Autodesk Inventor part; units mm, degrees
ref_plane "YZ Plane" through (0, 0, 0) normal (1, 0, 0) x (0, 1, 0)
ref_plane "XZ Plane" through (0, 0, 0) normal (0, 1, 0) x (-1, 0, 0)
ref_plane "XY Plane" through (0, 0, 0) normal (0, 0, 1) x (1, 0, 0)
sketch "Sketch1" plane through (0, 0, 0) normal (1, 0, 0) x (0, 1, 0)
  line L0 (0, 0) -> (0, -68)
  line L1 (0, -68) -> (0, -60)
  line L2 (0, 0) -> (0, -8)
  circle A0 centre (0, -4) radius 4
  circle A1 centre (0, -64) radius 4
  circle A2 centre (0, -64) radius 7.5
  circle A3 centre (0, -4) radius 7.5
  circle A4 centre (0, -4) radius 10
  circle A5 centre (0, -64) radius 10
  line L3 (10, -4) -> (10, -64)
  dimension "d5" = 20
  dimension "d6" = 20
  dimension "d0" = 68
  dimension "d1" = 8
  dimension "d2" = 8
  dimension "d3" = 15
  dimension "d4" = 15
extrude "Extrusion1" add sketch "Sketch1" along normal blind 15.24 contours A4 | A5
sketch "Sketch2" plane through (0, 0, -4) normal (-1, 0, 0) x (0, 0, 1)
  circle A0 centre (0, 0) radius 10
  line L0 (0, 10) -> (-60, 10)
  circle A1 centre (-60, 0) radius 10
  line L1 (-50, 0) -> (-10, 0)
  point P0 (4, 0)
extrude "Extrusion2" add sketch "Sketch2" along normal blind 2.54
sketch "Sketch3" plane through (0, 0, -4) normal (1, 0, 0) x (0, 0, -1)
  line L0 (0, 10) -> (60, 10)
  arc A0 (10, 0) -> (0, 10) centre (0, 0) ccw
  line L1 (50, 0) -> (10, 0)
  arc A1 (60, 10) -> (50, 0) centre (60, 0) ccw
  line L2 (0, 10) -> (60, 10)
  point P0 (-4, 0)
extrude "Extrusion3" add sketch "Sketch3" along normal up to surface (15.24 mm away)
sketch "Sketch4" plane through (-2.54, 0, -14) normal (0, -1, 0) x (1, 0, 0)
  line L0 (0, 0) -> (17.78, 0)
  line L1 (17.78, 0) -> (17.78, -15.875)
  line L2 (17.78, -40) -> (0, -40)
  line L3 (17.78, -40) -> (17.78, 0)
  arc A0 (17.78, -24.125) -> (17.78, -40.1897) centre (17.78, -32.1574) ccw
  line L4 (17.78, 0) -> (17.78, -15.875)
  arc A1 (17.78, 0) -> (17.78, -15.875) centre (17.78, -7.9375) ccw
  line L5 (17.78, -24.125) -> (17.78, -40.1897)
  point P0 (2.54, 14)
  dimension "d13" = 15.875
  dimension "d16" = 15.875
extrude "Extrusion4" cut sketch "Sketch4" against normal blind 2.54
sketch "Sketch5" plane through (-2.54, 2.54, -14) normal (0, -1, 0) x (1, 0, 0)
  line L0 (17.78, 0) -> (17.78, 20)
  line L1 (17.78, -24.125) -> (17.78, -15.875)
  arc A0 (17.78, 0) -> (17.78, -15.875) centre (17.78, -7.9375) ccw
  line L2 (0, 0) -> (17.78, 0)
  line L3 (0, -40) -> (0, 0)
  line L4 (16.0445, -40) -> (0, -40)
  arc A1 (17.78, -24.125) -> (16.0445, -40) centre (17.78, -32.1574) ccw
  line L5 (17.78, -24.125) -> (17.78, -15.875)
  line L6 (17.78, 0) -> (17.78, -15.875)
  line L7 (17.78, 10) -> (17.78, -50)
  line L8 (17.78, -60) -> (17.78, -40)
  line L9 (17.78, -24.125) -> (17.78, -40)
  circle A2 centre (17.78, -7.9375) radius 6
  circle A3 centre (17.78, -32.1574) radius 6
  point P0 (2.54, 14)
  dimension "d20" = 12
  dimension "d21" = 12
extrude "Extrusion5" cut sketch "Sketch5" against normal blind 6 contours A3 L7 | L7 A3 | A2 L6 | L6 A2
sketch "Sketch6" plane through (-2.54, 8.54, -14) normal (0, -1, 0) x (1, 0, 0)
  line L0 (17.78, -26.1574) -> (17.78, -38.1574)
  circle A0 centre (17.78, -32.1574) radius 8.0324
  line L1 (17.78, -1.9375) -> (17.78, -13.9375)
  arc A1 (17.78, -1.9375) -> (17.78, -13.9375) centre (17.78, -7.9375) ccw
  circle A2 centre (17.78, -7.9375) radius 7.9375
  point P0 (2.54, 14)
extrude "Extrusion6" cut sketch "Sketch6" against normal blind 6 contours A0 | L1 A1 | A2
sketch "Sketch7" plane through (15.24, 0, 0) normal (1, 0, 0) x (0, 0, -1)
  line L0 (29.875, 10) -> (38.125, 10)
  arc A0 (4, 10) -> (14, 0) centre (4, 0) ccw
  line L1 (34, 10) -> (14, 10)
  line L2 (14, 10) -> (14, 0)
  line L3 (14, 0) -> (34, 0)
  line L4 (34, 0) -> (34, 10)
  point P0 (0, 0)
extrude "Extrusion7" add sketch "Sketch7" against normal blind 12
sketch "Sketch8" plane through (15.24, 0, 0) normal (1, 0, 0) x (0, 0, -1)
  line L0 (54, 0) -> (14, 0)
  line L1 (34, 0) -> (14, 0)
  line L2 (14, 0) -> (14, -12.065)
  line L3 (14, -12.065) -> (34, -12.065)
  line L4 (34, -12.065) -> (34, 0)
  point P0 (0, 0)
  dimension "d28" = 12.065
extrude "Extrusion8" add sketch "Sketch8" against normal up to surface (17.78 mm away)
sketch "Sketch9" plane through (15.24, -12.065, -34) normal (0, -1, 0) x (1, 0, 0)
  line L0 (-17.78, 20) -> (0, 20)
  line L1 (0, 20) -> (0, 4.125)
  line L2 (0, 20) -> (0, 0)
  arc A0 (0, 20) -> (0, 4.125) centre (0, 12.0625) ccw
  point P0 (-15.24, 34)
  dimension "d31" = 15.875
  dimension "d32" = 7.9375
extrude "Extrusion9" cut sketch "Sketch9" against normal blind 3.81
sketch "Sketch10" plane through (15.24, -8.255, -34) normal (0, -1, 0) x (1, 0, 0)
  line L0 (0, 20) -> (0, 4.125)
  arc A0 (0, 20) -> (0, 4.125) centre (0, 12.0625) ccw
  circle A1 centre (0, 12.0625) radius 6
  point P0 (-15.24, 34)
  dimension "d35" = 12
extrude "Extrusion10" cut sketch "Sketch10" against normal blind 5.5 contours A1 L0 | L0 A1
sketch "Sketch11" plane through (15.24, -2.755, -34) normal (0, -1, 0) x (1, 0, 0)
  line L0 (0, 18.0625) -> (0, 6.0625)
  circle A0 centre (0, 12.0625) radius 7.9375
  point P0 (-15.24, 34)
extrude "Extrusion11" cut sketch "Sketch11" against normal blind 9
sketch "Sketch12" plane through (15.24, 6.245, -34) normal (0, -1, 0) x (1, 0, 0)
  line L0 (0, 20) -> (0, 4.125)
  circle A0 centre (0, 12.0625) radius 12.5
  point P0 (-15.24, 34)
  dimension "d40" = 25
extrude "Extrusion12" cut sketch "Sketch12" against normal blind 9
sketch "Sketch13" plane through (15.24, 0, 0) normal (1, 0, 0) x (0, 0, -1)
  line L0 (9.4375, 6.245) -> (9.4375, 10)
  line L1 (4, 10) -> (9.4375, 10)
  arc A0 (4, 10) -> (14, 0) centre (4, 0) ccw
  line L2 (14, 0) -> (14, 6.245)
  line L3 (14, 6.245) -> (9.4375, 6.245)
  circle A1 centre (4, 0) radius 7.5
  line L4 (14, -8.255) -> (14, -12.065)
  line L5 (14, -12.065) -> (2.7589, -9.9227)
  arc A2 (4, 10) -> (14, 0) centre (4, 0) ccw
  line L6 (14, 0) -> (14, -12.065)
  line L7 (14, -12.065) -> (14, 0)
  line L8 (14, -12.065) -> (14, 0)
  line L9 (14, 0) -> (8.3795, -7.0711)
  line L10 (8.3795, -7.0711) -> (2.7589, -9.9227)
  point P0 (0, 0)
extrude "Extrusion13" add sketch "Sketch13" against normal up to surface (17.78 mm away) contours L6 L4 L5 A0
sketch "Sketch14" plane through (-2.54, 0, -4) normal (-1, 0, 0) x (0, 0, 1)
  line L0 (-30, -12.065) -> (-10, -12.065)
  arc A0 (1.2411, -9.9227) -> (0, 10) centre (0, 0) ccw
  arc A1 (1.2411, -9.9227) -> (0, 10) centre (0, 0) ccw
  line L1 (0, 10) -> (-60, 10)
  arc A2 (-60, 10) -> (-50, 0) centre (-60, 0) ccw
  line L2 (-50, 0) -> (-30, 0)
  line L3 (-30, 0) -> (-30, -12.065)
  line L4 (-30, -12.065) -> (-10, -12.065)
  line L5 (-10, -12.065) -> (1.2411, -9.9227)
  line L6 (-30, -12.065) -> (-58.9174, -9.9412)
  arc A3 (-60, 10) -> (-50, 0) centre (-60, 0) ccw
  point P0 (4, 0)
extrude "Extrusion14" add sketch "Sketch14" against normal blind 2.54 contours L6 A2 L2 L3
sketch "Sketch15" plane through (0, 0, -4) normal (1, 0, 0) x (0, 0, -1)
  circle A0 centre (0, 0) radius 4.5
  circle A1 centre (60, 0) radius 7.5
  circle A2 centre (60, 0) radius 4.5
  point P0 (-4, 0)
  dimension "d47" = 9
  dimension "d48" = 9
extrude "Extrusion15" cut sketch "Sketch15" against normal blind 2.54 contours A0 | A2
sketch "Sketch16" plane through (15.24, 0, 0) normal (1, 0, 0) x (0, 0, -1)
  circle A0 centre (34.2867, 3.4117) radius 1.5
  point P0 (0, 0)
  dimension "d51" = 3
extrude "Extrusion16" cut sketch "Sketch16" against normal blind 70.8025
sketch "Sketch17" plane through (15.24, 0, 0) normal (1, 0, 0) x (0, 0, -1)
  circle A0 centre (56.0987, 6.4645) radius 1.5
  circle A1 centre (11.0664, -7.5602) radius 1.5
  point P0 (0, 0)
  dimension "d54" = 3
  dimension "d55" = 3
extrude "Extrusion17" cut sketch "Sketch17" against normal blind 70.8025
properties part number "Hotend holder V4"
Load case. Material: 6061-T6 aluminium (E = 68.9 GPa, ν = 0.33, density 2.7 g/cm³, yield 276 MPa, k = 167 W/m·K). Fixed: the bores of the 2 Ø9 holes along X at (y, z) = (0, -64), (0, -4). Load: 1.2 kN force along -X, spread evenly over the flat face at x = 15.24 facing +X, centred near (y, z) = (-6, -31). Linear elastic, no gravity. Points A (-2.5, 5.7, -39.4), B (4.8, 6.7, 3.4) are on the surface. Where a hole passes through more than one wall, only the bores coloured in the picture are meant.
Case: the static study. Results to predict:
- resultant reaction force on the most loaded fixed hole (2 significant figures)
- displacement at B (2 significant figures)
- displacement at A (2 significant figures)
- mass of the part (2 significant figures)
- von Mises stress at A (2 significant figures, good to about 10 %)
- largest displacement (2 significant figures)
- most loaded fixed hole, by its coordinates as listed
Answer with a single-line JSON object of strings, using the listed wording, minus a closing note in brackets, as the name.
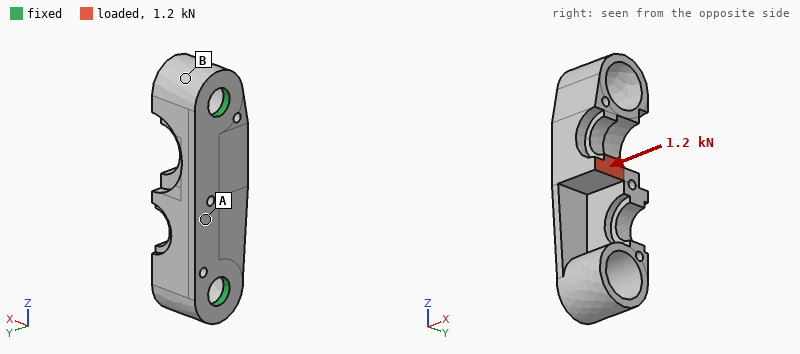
{"resultant reaction force on the most loaded fixed hole": "940 N", "displacement at B": "12 µm", "displacement at A": "16 µm", "mass of the part": "41 g", "von Mises stress at A": "22 MPa", "largest displacement": "63 µm", "most loaded fixed hole, by its coordinates as listed": "(0, -4)"}
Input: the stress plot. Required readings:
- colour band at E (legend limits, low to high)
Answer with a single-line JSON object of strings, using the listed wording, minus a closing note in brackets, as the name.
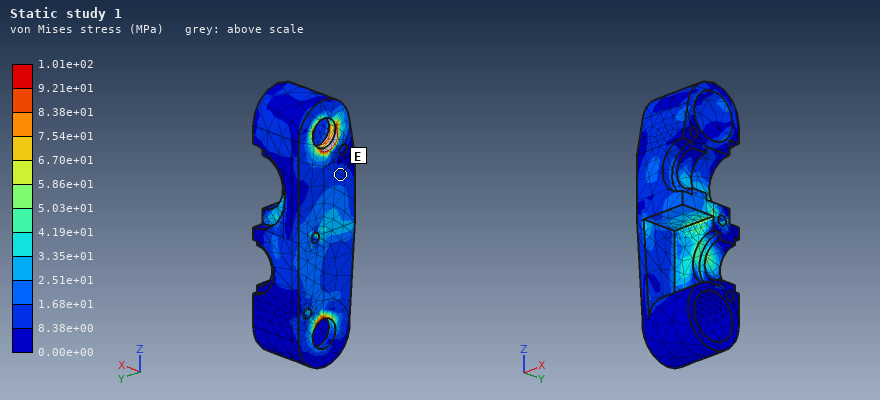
{"colour band at E": "8.38e+00 to 1.68e+01 MPa"}
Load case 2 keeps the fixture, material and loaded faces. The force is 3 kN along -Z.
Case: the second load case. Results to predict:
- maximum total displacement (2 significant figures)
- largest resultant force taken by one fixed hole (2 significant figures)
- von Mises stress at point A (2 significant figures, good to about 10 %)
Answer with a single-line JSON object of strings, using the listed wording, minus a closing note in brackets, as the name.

{"maximum total displacement": "99 µm", "largest resultant force taken by one fixed hole": "1.9 kN", "von Mises stress at point A": "36 MPa"}
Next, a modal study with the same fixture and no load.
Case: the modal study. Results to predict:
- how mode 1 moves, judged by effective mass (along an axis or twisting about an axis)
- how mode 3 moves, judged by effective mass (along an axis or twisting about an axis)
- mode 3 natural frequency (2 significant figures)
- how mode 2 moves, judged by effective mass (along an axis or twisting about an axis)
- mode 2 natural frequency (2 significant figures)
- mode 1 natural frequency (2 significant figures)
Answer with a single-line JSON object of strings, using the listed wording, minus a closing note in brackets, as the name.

{"how mode 1 moves, judged by effective mass": "along Y", "how mode 3 moves, judged by effective mass": "along Y", "mode 3 natural frequency": "14 kHz", "how mode 2 moves, judged by effective mass": "along X", "mode 2 natural frequency": "8000 Hz", "mode 1 natural frequency": "7000 Hz"}
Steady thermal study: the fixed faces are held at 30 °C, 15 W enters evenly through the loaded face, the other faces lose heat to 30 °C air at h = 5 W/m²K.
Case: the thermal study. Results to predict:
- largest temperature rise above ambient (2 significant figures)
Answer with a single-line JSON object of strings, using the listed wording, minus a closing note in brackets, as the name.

{"largest temperature rise above ambient": "20 K"}
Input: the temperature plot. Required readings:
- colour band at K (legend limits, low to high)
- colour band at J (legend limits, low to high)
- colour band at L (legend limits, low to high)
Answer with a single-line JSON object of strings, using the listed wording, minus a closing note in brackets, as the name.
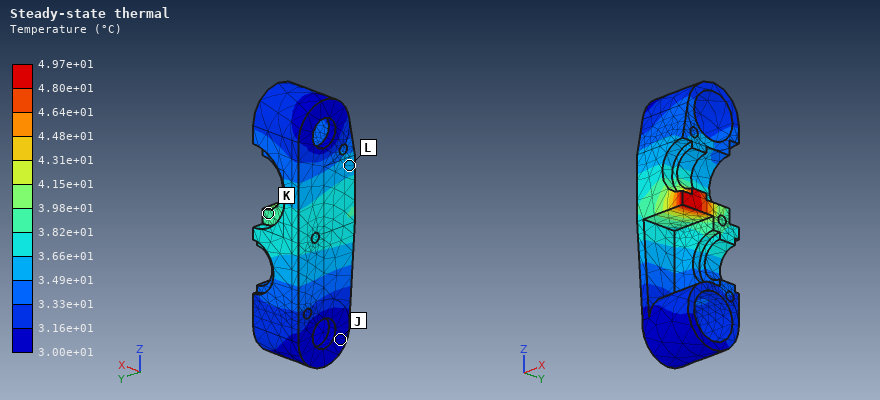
{"colour band at K": "3.82e+01 to 3.98e+01 °C", "colour band at J": "3.00e+01 to 3.16e+01 °C", "colour band at L": "3.49e+01 to 3.66e+01 °C"}
